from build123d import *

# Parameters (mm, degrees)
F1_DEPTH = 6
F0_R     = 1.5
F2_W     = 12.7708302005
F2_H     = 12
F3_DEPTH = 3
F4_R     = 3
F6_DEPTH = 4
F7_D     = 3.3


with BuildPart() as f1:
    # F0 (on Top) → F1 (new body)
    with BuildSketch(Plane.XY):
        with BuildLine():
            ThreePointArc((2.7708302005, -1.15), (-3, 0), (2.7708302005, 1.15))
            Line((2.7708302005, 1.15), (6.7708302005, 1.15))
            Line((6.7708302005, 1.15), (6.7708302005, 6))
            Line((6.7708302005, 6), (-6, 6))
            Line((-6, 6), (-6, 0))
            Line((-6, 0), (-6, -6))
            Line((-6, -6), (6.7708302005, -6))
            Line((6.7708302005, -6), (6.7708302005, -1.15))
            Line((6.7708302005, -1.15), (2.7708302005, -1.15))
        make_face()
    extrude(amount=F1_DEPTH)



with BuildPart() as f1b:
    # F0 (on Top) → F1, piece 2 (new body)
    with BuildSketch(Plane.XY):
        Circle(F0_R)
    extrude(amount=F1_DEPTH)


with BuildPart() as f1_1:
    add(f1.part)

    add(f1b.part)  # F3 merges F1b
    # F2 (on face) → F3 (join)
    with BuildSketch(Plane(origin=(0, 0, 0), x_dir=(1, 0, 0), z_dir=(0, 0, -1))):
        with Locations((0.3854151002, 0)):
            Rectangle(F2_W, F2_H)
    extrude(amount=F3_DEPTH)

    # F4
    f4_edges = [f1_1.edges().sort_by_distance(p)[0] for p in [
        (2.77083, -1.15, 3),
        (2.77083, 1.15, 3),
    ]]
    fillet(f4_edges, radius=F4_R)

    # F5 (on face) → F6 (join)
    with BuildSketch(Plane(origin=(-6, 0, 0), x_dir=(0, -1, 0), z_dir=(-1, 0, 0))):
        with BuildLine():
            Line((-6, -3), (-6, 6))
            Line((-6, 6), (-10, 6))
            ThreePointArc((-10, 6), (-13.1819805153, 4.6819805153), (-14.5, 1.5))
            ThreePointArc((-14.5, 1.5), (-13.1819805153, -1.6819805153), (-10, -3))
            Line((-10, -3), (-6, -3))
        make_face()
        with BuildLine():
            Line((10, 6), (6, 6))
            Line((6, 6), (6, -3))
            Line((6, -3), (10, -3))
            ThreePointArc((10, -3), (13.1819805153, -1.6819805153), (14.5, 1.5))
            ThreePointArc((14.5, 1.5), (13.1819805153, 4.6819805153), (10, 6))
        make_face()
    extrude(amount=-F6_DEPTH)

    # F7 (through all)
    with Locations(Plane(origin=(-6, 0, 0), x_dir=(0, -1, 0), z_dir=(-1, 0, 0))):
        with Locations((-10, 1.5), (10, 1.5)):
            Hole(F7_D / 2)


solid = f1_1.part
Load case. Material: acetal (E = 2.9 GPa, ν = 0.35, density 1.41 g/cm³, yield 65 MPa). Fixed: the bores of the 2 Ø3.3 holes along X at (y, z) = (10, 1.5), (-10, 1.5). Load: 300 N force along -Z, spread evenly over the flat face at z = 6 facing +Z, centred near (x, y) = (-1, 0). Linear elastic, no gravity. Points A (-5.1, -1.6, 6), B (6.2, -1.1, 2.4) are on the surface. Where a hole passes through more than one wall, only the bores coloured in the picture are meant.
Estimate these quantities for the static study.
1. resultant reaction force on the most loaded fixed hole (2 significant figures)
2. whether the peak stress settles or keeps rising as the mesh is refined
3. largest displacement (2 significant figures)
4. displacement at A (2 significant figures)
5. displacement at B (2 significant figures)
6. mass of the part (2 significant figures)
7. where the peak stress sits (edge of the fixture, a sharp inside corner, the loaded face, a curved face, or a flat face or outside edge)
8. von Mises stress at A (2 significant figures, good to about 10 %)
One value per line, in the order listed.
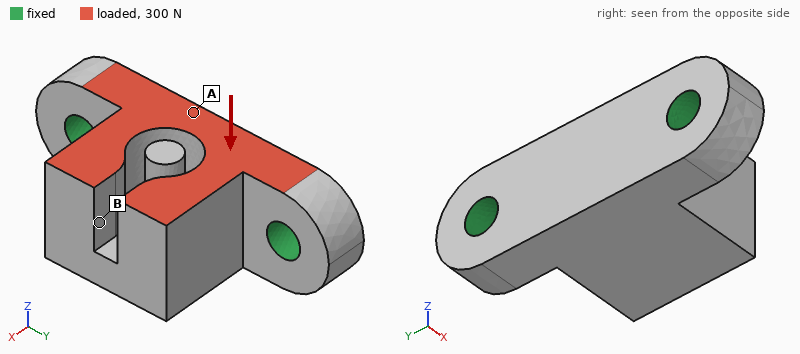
150 N
keeps rising
0.19 mm
0.053 mm
0.17 mm
2.4 g
edge of the fixture
7.6 MPa
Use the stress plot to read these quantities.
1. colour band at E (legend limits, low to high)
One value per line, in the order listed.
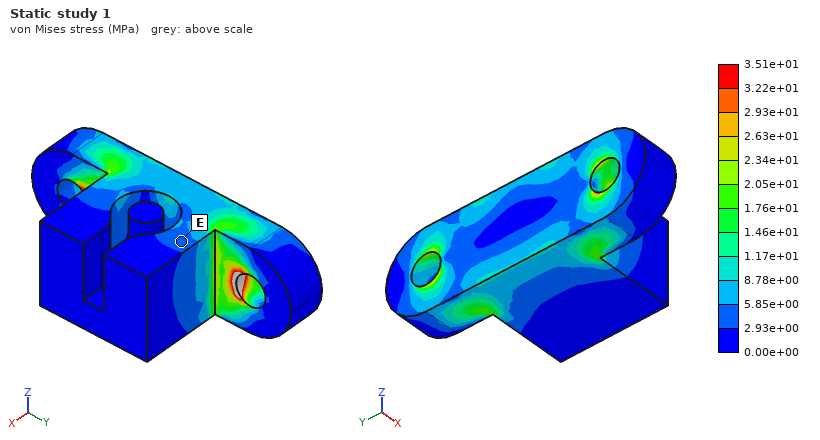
2.93e+00 to 5.85e+00 MPa
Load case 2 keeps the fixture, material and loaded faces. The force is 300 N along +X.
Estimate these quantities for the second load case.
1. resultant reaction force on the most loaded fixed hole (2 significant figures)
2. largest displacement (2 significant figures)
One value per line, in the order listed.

150 N
0.22 mm
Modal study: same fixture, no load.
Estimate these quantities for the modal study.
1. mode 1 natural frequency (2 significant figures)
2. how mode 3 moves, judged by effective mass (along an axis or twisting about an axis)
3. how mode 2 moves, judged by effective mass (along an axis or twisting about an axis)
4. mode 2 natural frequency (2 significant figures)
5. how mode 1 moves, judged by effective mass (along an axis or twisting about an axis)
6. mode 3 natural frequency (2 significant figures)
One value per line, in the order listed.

5000 Hz
along X
along Y
8700 Hz
along Z
9700 Hz
